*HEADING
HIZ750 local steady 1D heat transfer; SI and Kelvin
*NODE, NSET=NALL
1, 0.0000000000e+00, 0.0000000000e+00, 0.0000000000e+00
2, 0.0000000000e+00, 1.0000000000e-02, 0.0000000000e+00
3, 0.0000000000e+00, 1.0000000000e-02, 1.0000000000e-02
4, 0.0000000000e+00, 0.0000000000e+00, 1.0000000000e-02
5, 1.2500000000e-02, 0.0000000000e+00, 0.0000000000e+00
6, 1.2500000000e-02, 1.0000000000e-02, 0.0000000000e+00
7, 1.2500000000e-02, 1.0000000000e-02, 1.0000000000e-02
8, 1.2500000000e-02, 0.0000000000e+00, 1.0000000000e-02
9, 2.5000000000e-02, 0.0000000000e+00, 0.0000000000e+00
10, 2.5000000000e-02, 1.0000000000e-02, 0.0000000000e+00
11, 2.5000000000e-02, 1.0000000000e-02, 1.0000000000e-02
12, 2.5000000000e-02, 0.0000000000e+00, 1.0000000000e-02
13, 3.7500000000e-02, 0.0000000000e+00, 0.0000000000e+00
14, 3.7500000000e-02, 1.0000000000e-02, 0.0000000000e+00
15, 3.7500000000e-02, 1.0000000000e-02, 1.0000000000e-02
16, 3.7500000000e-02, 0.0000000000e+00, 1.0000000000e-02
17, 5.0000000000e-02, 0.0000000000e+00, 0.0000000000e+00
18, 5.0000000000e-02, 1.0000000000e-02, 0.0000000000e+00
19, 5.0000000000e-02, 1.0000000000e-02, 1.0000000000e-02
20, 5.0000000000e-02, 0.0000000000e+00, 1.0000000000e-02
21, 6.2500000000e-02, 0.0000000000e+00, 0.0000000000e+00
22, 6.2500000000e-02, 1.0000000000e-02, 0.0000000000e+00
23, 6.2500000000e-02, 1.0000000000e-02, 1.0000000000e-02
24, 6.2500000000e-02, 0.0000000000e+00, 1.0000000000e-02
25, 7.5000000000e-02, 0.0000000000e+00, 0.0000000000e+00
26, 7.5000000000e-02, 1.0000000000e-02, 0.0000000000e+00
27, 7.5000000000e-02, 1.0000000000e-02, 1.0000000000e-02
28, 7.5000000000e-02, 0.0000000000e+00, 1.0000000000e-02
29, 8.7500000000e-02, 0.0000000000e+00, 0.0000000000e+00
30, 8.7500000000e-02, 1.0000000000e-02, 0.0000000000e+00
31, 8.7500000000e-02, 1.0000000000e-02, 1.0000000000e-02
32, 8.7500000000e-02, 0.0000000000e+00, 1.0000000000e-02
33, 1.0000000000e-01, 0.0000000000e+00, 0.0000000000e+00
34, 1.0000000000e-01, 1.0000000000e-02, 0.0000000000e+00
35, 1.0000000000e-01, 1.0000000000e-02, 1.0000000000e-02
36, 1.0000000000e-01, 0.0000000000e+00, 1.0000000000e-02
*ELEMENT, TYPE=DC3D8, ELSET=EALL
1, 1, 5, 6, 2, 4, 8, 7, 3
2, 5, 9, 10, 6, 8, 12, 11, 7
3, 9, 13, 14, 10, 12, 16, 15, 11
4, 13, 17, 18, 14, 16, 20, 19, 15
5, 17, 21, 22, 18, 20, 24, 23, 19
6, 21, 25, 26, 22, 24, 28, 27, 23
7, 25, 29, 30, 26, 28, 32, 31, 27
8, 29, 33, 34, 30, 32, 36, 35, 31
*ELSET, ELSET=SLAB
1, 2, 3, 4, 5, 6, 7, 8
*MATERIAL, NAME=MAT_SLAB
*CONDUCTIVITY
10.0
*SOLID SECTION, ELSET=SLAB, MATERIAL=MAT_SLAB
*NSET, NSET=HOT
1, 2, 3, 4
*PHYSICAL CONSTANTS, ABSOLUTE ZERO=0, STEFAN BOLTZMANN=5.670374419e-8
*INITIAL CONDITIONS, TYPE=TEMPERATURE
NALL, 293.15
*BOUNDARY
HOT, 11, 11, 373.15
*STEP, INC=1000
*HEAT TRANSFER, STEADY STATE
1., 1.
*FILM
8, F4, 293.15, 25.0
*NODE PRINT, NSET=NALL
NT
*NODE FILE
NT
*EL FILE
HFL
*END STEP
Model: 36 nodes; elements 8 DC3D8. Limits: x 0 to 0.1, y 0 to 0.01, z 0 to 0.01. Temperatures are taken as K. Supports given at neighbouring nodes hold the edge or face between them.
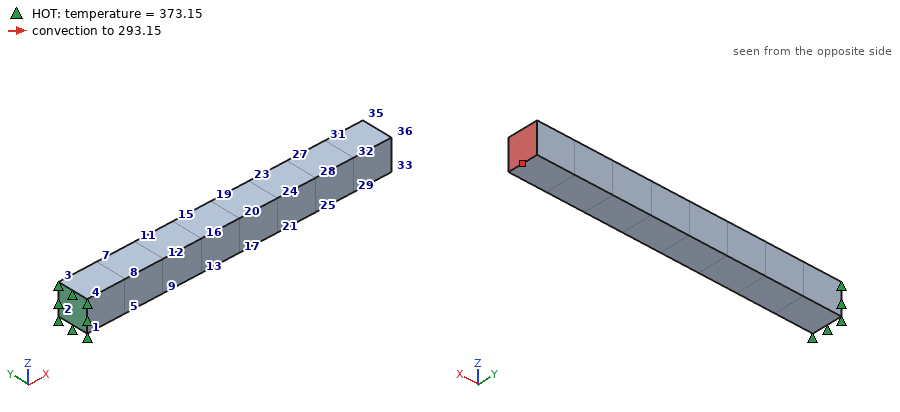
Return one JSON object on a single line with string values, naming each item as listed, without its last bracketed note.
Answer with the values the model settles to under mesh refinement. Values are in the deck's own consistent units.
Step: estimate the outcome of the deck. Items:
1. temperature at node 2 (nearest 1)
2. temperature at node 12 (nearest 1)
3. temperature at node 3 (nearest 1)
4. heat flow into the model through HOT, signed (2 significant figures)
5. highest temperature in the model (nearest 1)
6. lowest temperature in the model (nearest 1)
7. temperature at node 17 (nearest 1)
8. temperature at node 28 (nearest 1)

{"temperature at node 2": "373 K", "temperature at node 12": "369 K", "temperature at node 3": "373 K", "heat flow into the model through HOT, signed": "0.16", "highest temperature in the model": "373 K", "lowest temperature in the model": "357 K", "temperature at node 17": "365 K", "temperature at node 28": "361 K"}
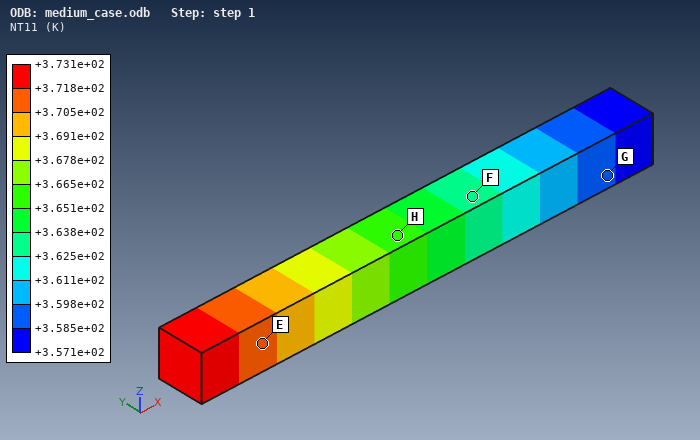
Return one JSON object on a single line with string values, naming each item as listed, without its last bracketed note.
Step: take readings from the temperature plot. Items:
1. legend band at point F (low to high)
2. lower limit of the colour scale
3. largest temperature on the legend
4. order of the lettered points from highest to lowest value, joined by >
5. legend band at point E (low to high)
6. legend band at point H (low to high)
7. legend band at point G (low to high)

{"legend band at point F": "+3.625e+02 to +3.638e+02 K", "lower limit of the colour scale": "+3.571e+02 K", "largest temperature on the legend": "+3.731e+02 K", "order of the lettered points from highest to lowest value, joined by >": "E > H > F > G", "legend band at point E": "+3.705e+02 to +3.718e+02 K", "legend band at point H": "+3.651e+02 to +3.665e+02 K", "legend band at point G": "+3.585e+02 to +3.598e+02 K"}
